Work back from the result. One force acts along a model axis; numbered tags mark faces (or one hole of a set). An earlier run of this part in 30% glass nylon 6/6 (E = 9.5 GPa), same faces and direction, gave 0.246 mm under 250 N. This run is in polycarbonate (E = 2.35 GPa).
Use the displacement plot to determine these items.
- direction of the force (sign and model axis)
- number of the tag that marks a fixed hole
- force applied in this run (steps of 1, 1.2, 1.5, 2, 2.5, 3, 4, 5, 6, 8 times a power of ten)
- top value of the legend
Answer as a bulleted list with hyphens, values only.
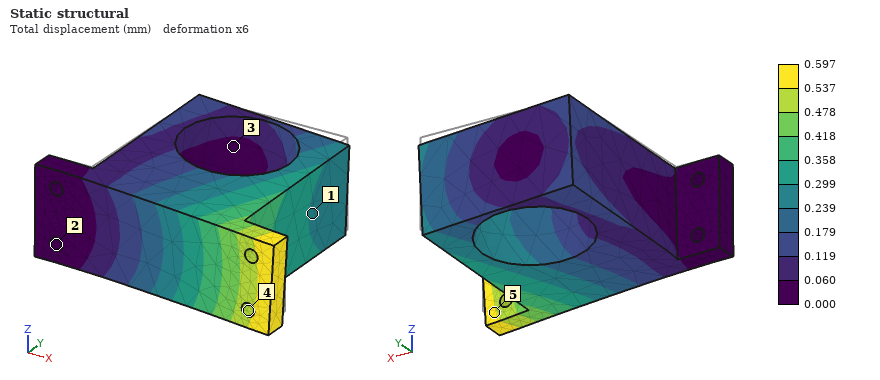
- -Z
- 2
- 150 N
- 0.597 mm
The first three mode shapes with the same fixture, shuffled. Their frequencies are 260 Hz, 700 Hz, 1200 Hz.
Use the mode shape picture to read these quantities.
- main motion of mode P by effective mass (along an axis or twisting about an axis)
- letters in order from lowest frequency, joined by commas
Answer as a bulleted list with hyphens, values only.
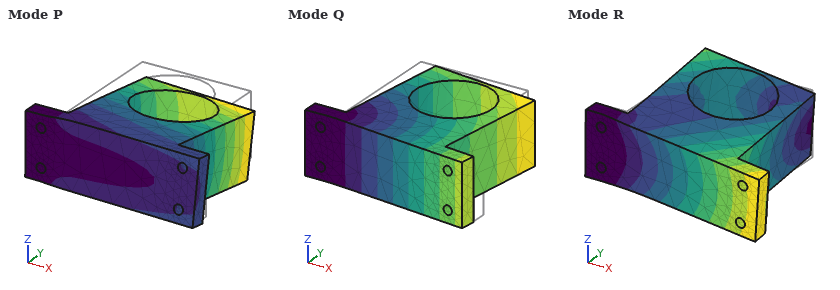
- along Z
- Q, P, R
